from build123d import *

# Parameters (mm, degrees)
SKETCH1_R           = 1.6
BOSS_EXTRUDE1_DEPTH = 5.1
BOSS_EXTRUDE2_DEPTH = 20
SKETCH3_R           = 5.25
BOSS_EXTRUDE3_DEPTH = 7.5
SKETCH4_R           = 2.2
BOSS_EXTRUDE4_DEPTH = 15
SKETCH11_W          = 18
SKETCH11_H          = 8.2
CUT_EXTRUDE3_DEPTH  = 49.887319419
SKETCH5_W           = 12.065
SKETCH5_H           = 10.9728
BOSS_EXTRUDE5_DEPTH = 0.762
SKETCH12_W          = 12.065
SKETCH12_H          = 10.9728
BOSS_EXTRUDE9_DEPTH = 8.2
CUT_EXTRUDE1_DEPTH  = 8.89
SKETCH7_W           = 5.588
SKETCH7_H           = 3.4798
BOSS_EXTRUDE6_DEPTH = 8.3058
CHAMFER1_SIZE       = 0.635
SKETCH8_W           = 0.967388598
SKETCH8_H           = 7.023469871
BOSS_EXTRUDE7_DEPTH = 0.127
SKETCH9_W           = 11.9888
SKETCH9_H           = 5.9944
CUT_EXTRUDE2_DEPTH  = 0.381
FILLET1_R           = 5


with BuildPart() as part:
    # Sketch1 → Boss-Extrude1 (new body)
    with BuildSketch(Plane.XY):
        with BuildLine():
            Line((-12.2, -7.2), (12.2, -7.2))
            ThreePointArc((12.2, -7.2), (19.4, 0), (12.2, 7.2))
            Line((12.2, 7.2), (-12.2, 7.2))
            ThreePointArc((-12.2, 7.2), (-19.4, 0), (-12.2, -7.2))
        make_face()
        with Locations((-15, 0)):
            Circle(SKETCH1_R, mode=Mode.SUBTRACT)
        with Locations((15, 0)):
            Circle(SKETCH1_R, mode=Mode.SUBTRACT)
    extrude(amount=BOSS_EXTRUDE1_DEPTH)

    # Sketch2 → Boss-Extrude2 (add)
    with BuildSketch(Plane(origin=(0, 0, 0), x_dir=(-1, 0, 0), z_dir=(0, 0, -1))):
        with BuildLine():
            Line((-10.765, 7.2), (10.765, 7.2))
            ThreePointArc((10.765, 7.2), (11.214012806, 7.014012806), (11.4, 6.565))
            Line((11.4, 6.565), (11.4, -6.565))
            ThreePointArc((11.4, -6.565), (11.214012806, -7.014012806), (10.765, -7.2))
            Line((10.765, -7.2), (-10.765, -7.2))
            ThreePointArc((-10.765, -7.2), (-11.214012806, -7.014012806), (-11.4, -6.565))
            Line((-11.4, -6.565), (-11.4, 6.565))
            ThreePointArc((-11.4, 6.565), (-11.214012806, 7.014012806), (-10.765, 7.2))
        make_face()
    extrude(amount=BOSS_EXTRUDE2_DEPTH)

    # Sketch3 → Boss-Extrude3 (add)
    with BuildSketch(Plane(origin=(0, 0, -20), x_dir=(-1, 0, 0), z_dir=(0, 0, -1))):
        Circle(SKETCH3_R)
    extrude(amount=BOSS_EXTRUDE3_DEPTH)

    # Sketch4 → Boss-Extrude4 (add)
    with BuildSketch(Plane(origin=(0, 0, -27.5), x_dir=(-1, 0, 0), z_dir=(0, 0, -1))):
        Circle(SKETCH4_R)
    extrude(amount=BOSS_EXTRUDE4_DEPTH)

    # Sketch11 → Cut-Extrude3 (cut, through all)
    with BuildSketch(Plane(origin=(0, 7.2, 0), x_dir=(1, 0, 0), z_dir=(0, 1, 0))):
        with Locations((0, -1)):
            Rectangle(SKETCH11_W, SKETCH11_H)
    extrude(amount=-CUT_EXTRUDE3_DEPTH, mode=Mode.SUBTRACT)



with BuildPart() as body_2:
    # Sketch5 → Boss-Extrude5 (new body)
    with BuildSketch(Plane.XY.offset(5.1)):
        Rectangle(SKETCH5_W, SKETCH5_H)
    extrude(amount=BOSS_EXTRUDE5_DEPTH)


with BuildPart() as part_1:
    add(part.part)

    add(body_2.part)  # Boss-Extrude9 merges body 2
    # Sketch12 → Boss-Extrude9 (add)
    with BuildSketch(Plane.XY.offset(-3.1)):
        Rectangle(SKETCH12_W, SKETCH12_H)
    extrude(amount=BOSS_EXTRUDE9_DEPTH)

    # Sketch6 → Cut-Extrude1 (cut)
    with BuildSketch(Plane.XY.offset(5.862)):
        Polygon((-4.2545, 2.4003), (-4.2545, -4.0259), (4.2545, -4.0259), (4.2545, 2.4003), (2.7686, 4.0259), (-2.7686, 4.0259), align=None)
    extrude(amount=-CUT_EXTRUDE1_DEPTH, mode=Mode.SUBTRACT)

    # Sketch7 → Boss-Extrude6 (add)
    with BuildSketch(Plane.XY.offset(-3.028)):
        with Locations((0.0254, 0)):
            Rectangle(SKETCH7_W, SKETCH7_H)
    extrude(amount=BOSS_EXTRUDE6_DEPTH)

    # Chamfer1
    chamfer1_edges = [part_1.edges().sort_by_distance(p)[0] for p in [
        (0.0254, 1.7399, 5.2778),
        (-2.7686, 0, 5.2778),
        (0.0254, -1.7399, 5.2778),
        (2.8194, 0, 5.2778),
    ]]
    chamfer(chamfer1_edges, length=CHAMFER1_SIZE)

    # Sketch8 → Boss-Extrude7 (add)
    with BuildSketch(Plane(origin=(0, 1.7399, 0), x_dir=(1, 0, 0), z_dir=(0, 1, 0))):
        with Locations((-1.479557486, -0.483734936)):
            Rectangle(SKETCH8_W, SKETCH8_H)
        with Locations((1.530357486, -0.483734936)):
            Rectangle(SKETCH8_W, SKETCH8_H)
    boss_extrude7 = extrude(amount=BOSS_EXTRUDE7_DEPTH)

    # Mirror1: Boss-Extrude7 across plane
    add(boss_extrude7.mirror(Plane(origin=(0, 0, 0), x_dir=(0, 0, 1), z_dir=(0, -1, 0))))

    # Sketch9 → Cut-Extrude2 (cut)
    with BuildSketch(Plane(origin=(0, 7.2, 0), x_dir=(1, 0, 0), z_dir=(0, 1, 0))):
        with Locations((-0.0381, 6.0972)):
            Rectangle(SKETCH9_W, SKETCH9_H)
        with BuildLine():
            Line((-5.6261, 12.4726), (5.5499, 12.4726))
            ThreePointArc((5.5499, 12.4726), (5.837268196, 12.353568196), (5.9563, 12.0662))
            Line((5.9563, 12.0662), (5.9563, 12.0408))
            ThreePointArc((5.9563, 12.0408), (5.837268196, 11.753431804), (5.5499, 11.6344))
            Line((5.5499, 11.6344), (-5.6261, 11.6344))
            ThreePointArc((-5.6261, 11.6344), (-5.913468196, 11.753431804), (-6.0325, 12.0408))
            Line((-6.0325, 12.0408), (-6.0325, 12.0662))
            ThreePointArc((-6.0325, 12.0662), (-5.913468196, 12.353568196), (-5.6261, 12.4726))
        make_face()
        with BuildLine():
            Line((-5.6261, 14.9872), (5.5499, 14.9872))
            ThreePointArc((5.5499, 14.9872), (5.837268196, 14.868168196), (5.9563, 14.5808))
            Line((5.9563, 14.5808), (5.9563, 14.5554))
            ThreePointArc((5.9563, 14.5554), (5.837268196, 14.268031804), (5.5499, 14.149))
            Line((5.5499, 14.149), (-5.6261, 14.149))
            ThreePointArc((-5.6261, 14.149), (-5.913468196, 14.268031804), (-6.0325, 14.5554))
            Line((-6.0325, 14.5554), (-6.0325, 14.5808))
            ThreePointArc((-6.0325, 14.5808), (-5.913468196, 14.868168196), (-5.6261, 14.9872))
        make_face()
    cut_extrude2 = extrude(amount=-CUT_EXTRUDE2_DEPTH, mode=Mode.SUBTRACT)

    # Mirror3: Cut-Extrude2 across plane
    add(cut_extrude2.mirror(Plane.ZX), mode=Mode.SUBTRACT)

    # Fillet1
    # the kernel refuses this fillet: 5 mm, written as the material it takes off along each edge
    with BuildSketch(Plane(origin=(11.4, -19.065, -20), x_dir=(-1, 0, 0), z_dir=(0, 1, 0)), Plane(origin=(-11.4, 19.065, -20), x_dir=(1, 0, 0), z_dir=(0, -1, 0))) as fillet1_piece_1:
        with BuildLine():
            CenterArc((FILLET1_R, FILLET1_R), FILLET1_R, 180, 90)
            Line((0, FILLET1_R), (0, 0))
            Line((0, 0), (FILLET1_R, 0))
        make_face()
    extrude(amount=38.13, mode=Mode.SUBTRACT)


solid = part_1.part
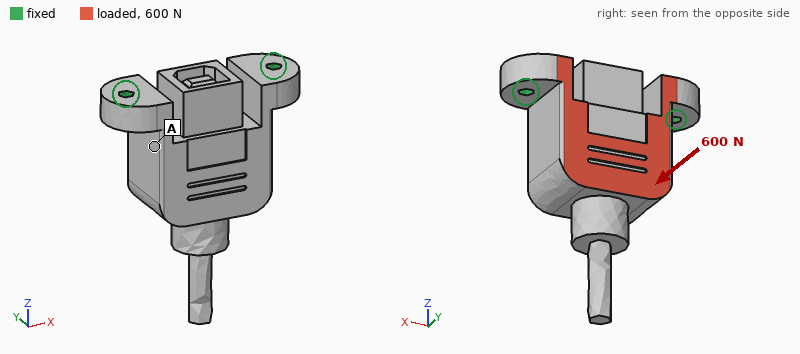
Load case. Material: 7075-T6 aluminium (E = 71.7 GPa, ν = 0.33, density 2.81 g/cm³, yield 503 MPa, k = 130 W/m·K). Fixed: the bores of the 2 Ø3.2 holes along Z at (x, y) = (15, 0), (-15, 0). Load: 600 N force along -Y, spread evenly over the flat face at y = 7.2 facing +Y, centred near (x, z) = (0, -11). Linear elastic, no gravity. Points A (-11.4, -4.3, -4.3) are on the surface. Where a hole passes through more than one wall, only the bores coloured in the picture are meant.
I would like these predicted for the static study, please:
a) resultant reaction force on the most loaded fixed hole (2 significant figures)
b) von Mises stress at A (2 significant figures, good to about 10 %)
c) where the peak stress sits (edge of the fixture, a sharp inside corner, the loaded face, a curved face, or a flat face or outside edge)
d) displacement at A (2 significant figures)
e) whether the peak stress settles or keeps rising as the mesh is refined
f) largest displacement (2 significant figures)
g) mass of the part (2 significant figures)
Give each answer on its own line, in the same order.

300 N
18 MPa
edge of the fixture
15 µm
keeps rising
87 µm
24 g
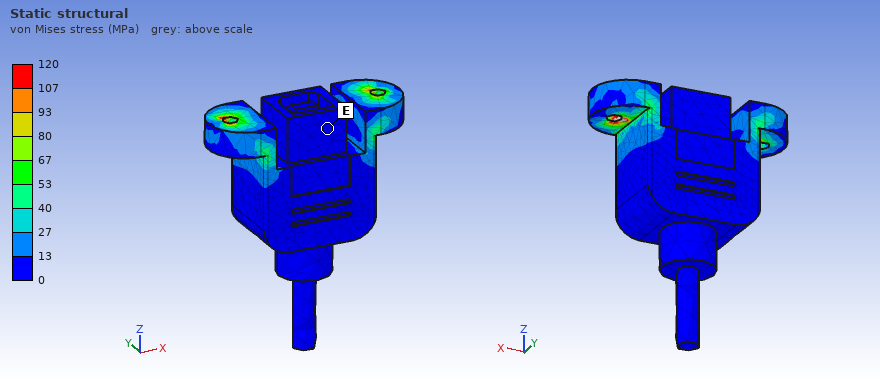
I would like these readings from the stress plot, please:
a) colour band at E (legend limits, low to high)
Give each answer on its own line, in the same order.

0 to 13 MPa
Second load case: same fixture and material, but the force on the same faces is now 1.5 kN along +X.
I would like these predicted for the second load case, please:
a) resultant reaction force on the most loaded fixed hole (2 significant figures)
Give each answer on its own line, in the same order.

1.1 kN
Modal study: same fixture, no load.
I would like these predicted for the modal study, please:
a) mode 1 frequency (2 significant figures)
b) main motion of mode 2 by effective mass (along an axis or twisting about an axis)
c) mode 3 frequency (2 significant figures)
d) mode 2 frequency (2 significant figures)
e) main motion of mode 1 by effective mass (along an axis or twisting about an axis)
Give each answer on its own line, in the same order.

4200 Hz
along X
12 kHz
9800 Hz
along Y
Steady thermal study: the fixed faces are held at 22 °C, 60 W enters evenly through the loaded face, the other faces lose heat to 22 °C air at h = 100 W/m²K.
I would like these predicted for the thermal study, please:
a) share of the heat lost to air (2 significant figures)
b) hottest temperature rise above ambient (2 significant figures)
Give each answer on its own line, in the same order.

22 %
55 K
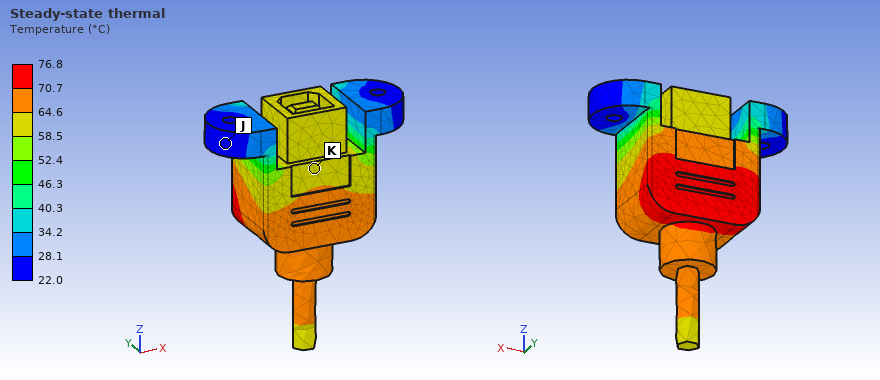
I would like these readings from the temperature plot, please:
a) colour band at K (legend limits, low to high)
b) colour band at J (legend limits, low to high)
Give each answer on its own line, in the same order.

58.5 to 64.6 °C
22.0 to 28.1 °C
